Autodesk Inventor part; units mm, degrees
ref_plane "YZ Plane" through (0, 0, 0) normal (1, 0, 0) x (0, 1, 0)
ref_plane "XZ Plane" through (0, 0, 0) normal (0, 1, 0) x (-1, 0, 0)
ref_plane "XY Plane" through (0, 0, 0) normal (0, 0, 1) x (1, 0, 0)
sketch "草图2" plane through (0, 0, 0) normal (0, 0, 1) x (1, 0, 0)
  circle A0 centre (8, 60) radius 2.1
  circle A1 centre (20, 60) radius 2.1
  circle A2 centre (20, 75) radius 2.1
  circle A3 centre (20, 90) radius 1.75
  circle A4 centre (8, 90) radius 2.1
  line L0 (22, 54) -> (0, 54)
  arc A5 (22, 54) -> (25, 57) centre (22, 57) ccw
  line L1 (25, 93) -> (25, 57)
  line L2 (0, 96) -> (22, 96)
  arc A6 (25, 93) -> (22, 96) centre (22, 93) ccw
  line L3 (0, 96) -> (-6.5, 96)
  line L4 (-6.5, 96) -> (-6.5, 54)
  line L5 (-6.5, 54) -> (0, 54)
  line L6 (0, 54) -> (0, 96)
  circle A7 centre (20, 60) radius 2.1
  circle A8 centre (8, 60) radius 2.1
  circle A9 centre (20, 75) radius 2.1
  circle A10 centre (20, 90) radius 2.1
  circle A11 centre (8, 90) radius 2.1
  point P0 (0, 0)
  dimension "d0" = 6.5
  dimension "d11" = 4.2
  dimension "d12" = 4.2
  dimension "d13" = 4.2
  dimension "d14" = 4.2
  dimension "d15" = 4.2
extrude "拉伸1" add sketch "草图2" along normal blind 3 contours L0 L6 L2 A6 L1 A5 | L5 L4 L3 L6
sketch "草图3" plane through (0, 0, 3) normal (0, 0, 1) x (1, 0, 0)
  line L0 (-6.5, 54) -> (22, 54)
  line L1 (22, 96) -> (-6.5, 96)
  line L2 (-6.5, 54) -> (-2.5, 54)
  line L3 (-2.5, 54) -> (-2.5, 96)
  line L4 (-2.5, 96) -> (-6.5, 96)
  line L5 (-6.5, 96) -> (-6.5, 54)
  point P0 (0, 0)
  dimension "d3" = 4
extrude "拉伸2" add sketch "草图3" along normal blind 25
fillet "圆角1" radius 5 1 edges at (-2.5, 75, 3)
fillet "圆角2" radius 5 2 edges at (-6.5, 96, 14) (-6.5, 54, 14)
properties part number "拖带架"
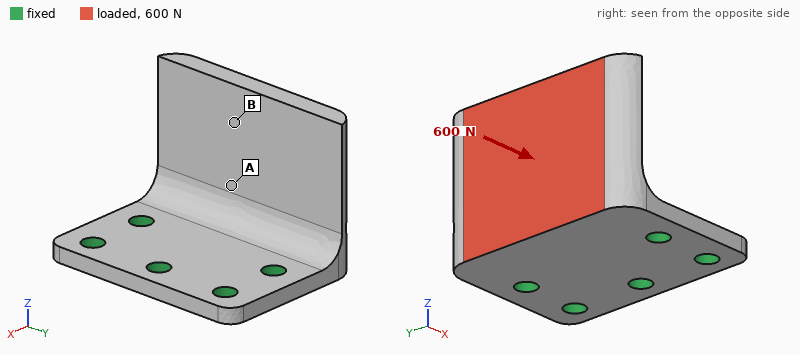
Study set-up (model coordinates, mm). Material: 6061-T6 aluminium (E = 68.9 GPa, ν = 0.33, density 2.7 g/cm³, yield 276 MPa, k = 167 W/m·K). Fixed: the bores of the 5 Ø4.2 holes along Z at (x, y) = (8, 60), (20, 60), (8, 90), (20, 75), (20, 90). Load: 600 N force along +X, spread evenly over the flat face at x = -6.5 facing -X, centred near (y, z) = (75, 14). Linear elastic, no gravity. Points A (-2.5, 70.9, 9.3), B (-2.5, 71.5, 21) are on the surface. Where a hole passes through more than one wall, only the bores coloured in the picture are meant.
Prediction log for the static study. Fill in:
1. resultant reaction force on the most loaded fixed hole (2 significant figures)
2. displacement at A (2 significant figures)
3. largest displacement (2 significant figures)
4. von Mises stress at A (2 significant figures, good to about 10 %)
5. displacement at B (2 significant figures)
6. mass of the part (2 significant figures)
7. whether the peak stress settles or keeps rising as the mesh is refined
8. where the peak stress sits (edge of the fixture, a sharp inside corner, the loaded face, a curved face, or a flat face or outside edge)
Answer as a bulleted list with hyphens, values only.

- 240 N
- 0.093 mm
- 0.32 mm
- 39 MPa
- 0.22 mm
- 21 g
- keeps rising
- edge of the fixture
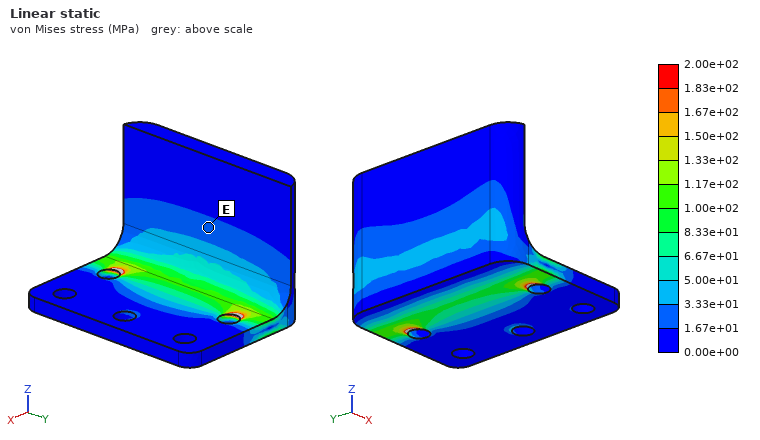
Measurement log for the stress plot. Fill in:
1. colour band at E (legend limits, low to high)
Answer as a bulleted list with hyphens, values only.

- 1.67e+01 to 3.33e+01 MPa
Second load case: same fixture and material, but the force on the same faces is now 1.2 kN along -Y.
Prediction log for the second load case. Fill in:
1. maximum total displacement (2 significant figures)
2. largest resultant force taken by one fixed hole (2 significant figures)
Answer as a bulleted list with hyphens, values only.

- 74 µm
- 880 N
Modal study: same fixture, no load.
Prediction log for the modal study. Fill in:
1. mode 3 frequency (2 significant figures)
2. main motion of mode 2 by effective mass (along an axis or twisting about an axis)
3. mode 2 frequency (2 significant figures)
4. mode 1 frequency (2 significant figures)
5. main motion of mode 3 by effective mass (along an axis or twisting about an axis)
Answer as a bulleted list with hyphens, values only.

- 8700 Hz
- along Y
- 5400 Hz
- 2300 Hz
- along Z
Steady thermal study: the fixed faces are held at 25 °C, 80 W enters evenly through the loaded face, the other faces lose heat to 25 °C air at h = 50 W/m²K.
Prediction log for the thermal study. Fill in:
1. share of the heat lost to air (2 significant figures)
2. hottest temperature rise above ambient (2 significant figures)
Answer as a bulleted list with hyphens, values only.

- 7.8 %
- 74 K
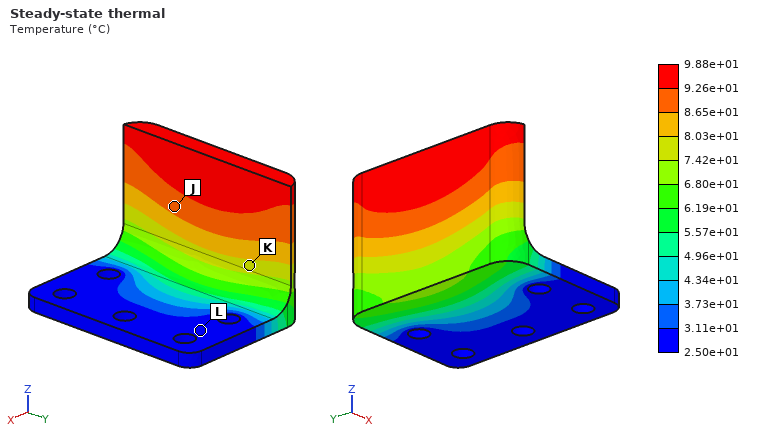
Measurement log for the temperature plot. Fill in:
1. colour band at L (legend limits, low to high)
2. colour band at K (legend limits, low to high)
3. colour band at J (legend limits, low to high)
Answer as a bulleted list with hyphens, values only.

- 2.50e+01 to 3.11e+01 °C
- 7.42e+01 to 8.03e+01 °C
- 8.65e+01 to 9.26e+01 °C
